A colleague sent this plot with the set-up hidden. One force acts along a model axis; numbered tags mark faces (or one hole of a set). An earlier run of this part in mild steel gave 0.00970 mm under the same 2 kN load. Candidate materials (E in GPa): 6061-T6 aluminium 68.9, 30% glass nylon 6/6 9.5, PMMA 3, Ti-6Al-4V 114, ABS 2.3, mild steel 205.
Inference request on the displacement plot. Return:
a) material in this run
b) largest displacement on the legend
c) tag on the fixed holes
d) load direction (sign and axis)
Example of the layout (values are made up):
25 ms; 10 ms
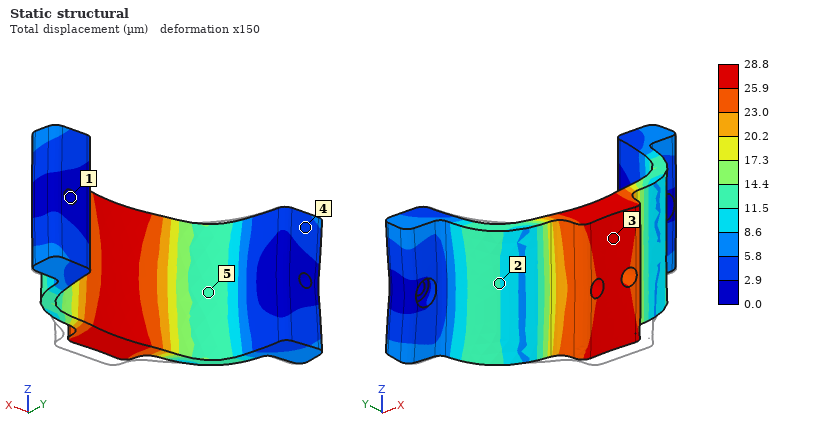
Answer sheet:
6061-T6 aluminium; 28.8 µm; 1; +Y
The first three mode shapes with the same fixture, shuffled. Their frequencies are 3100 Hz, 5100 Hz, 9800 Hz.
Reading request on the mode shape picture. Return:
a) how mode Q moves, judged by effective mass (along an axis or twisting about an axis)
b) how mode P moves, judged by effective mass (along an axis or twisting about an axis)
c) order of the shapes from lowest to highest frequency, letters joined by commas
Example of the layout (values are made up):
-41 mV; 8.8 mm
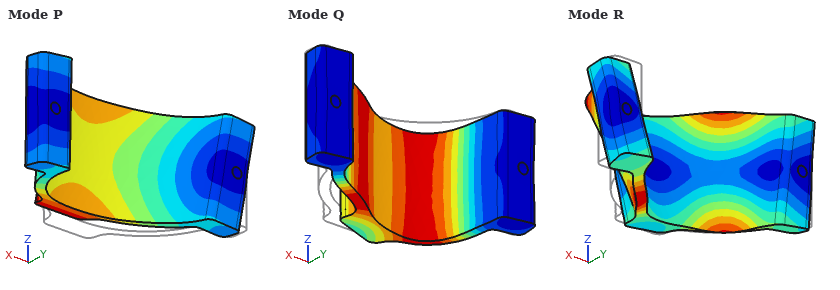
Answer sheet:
along X; along Z; P, Q, R
